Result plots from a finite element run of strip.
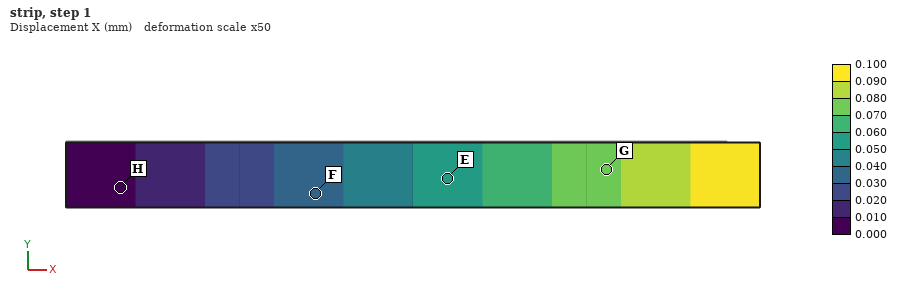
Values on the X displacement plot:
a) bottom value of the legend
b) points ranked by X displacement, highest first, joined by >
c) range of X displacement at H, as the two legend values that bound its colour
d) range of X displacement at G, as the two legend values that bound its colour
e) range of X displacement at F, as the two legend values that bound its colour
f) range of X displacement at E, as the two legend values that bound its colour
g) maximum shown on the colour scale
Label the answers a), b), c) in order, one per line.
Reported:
a) 0.000 mm
b) G > E > F > H
c) 0.000 to 0.010 mm
d) 0.070 to 0.080 mm
e) 0.030 to 0.040 mm
f) 0.050 to 0.060 mm
g) 0.100 mm
